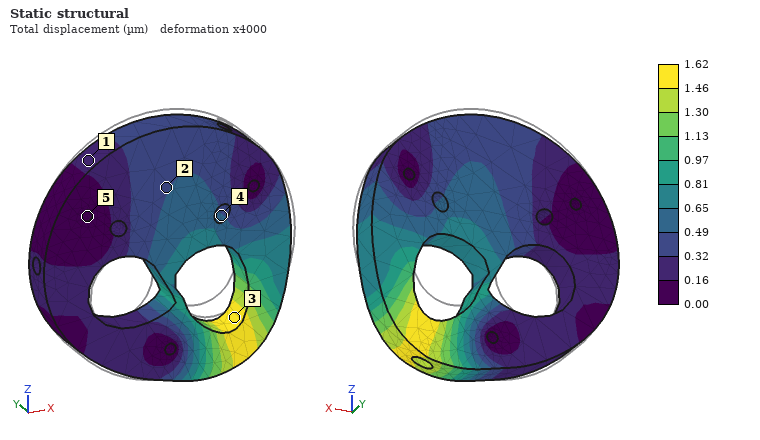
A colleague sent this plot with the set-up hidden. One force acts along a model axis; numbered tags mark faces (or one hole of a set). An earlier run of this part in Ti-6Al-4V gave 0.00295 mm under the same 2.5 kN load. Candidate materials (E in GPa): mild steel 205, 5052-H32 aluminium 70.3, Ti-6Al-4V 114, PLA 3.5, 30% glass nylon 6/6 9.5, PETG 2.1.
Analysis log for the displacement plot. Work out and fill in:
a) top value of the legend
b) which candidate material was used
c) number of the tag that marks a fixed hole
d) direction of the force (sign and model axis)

1.62 µm
mild steel
5
-Z
